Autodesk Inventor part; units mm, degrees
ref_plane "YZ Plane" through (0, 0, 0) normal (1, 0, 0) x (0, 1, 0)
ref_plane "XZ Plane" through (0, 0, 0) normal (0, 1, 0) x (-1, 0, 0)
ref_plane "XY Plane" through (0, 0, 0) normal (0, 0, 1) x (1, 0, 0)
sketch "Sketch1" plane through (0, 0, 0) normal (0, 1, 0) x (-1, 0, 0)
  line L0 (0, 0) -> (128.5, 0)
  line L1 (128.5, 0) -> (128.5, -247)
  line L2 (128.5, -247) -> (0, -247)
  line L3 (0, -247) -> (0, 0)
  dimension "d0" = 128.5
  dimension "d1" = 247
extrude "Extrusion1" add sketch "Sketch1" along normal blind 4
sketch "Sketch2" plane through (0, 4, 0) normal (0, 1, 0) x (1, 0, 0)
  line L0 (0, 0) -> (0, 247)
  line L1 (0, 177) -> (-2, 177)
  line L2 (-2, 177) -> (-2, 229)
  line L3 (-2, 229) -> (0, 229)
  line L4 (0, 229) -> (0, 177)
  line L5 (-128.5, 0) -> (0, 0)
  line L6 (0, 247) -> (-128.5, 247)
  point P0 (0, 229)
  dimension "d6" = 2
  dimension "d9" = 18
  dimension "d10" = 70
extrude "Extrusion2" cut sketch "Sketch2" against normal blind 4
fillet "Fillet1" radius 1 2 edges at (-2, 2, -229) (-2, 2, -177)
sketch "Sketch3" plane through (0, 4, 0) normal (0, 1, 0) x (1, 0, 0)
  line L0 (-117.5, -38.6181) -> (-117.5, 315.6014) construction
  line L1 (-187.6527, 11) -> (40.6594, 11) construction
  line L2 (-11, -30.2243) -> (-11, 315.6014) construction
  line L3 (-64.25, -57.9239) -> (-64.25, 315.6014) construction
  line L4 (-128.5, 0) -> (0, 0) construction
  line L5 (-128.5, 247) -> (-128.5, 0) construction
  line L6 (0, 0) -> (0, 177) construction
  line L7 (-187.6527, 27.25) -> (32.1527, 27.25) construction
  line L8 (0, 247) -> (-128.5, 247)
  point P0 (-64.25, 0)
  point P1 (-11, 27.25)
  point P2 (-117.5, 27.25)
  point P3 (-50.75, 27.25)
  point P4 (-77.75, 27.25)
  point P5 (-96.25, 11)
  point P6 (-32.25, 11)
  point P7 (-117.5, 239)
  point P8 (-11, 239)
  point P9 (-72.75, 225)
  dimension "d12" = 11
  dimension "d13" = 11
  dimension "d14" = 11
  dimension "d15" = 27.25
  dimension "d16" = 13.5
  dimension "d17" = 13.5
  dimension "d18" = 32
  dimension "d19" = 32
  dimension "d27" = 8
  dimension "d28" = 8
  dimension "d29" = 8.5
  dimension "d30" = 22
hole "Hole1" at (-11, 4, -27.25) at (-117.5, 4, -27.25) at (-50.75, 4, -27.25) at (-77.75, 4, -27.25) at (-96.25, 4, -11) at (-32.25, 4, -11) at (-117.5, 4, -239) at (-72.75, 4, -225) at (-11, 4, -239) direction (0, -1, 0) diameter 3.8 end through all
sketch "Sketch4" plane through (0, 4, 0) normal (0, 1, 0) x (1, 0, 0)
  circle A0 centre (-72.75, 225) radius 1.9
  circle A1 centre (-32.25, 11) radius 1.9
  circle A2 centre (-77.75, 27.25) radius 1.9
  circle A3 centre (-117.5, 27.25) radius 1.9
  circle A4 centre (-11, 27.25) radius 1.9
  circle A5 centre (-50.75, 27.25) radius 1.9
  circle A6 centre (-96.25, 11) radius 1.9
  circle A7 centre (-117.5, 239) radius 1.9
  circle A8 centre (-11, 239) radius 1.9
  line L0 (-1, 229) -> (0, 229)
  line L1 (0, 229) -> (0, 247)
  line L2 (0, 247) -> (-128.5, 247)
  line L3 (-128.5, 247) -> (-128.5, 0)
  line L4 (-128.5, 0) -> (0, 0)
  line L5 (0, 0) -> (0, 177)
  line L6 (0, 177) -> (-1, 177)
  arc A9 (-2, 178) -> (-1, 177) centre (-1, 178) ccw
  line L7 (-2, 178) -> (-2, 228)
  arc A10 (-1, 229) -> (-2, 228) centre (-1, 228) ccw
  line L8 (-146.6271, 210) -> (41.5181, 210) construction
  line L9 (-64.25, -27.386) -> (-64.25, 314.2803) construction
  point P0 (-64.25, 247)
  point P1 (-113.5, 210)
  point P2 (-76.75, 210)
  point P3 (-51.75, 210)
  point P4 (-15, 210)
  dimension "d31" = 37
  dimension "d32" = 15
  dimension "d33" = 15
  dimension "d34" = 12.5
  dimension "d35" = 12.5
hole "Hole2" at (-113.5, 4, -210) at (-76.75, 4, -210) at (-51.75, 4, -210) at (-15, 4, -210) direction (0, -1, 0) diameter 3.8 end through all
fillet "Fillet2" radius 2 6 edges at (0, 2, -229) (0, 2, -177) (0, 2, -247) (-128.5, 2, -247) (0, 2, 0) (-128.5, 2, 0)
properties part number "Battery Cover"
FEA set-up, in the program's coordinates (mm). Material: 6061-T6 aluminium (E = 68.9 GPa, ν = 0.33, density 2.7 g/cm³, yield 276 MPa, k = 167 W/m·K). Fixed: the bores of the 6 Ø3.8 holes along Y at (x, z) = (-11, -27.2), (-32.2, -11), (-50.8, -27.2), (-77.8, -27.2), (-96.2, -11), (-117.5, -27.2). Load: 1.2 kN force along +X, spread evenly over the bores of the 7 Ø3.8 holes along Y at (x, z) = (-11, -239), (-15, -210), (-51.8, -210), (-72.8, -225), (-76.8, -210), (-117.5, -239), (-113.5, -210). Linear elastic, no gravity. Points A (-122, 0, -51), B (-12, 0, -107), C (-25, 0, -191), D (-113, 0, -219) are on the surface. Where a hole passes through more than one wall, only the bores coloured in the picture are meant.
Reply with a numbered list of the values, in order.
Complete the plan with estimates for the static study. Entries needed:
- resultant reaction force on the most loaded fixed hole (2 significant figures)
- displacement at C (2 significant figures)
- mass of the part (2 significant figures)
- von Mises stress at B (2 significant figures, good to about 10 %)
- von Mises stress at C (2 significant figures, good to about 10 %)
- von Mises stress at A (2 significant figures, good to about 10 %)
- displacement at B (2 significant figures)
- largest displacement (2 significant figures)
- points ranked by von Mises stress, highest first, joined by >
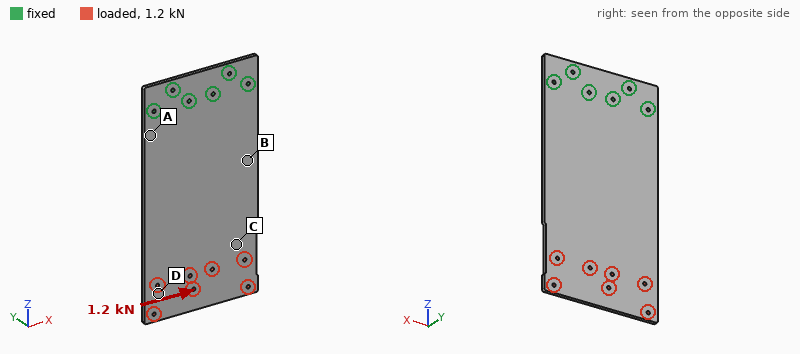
1. 1.8 kN
2. 0.072 mm
3. 340 g
4. 10 MPa
5. 4.4 MPa
6. 17 MPa
7. 0.031 mm
8. 0.11 mm
9. A > B > C > D
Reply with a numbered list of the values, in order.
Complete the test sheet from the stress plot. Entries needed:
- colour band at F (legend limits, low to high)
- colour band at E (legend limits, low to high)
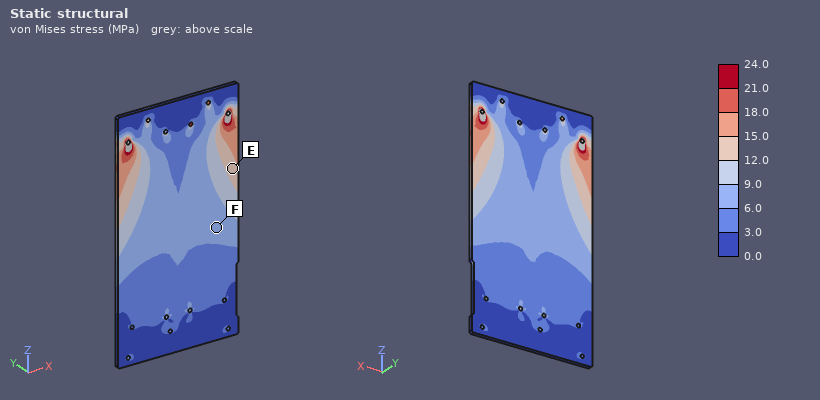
1. 6.0 to 9.0 MPa
2. 12.0 to 15.0 MPa
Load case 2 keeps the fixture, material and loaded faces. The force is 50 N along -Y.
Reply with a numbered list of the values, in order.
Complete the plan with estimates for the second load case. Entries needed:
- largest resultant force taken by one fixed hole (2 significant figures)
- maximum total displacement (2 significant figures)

1. 87 N
2. 3.0 mm
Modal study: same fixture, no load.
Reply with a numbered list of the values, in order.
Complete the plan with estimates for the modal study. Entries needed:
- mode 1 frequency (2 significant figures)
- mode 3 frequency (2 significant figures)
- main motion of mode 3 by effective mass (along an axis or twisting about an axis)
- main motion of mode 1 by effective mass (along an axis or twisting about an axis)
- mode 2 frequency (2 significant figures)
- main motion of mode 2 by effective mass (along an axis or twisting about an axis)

1. 69 Hz
2. 430 Hz
3. along Y
4. along Y
5. 260 Hz
6. twisting about Z
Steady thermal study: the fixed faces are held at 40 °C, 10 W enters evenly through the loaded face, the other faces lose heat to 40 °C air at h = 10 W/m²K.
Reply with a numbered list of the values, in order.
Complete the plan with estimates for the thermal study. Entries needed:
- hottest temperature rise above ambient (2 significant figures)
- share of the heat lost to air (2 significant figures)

1. 16 K
2. 46 %
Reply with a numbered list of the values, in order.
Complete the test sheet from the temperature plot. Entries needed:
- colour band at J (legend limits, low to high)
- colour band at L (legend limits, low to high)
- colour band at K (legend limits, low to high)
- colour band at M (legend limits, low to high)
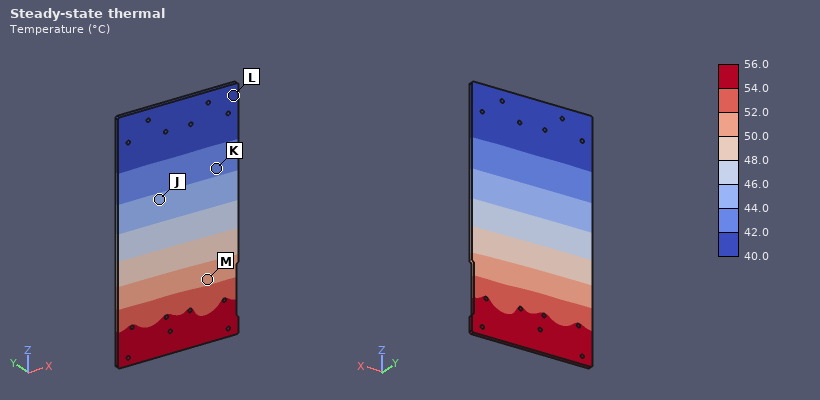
1. 44.0 to 46.0 °C
2. 40.0 to 42.0 °C
3. 42.0 to 44.0 °C
4. 50.0 to 52.0 °C
